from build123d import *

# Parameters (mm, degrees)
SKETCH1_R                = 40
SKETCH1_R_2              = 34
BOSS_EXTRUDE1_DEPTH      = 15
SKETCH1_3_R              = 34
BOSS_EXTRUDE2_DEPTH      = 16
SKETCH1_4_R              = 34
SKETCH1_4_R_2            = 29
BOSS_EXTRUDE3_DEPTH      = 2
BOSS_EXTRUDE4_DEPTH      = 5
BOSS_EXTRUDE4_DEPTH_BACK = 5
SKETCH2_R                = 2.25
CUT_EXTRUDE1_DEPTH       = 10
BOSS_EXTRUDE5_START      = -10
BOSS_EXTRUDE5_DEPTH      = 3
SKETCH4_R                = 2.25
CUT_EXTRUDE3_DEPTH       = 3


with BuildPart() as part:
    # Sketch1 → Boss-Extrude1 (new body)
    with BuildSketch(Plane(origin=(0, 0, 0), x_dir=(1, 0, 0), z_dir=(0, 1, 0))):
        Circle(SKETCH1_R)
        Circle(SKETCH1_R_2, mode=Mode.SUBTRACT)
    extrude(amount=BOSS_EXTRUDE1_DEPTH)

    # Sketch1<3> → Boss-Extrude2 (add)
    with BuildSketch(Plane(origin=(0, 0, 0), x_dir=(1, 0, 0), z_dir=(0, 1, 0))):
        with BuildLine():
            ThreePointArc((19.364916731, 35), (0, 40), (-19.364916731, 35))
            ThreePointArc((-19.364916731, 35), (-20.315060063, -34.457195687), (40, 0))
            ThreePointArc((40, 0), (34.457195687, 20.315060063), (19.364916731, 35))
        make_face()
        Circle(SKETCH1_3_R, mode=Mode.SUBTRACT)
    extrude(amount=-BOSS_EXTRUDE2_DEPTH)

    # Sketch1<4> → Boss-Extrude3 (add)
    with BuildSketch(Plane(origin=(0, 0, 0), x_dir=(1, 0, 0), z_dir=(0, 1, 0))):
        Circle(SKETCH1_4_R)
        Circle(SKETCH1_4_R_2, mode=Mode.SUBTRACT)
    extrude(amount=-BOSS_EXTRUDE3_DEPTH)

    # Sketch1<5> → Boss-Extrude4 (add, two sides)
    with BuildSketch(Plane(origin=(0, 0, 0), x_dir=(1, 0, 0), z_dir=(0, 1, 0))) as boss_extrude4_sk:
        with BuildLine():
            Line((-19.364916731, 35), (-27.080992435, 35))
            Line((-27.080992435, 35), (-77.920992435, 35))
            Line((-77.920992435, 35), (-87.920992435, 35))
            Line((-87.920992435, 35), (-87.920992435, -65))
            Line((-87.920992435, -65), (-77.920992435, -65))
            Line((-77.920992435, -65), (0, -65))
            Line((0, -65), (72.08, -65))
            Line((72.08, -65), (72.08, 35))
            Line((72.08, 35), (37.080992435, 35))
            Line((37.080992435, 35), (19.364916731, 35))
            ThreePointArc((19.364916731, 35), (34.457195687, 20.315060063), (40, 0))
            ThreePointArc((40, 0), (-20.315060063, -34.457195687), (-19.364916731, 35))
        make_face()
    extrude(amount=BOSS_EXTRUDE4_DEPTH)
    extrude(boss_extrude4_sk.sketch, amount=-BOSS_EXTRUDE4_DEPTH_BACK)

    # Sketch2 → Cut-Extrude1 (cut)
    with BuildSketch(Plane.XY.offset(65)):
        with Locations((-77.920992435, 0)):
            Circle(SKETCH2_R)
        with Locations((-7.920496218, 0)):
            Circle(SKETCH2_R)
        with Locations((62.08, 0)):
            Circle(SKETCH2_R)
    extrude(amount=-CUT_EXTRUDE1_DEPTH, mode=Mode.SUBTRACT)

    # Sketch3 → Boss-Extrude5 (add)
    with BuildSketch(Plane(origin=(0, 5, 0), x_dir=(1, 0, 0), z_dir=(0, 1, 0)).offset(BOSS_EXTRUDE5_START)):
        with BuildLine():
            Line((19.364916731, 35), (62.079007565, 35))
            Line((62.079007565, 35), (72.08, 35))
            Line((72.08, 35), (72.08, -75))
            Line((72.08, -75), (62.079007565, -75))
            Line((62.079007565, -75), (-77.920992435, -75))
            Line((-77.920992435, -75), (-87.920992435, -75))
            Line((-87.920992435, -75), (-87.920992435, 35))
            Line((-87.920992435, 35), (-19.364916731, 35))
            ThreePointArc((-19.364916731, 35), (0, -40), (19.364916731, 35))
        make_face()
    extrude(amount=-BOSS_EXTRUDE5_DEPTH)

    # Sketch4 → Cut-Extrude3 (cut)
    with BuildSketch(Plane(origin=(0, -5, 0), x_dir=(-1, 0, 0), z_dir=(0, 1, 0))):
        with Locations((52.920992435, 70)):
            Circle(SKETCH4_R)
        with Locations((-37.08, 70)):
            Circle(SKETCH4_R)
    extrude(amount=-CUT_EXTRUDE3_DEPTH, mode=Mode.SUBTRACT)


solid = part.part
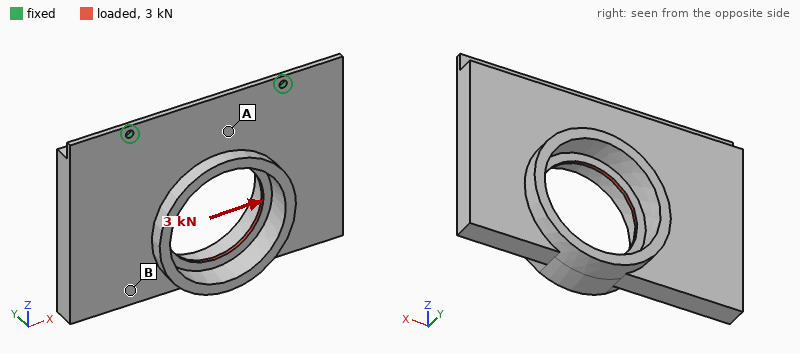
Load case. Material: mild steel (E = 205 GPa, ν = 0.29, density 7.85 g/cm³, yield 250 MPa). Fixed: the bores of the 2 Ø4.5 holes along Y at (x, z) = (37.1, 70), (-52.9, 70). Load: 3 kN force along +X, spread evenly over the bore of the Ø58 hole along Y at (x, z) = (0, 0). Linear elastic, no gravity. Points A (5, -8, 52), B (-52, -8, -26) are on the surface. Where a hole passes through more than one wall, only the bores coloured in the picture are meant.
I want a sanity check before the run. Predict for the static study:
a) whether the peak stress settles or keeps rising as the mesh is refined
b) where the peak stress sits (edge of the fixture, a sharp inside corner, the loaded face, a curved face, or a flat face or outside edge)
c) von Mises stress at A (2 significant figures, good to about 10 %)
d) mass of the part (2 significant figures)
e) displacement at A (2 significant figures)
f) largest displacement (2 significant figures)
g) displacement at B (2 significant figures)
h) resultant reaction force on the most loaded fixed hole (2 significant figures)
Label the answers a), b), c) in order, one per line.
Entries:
a) keeps rising
b) edge of the fixture
c) 15 MPa
d) 1.5 kg
e) 4.6 µm
f) 25 µm
g) 19 µm
h) 2.8 kN
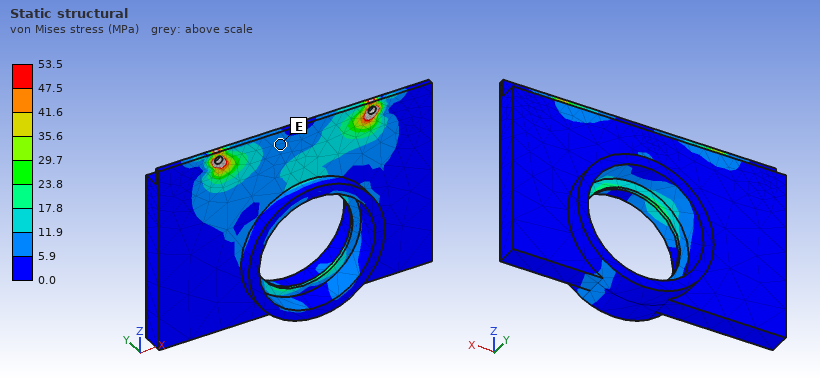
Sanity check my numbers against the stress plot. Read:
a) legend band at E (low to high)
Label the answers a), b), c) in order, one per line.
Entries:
a) 5.9 to 11.9 MPa
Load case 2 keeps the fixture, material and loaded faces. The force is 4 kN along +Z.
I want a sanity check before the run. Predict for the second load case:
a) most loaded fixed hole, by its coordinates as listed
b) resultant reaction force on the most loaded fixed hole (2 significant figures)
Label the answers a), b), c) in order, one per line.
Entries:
a) (37.1, 70)
b) 2.3 kN
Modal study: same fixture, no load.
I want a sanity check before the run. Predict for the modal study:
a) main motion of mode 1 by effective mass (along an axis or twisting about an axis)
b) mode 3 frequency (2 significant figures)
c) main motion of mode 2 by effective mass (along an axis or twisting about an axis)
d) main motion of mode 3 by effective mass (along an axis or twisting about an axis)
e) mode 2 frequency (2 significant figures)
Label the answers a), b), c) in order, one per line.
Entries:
a) along Y
b) 2200 Hz
c) twisting about Z
d) along X
e) 950 Hz
